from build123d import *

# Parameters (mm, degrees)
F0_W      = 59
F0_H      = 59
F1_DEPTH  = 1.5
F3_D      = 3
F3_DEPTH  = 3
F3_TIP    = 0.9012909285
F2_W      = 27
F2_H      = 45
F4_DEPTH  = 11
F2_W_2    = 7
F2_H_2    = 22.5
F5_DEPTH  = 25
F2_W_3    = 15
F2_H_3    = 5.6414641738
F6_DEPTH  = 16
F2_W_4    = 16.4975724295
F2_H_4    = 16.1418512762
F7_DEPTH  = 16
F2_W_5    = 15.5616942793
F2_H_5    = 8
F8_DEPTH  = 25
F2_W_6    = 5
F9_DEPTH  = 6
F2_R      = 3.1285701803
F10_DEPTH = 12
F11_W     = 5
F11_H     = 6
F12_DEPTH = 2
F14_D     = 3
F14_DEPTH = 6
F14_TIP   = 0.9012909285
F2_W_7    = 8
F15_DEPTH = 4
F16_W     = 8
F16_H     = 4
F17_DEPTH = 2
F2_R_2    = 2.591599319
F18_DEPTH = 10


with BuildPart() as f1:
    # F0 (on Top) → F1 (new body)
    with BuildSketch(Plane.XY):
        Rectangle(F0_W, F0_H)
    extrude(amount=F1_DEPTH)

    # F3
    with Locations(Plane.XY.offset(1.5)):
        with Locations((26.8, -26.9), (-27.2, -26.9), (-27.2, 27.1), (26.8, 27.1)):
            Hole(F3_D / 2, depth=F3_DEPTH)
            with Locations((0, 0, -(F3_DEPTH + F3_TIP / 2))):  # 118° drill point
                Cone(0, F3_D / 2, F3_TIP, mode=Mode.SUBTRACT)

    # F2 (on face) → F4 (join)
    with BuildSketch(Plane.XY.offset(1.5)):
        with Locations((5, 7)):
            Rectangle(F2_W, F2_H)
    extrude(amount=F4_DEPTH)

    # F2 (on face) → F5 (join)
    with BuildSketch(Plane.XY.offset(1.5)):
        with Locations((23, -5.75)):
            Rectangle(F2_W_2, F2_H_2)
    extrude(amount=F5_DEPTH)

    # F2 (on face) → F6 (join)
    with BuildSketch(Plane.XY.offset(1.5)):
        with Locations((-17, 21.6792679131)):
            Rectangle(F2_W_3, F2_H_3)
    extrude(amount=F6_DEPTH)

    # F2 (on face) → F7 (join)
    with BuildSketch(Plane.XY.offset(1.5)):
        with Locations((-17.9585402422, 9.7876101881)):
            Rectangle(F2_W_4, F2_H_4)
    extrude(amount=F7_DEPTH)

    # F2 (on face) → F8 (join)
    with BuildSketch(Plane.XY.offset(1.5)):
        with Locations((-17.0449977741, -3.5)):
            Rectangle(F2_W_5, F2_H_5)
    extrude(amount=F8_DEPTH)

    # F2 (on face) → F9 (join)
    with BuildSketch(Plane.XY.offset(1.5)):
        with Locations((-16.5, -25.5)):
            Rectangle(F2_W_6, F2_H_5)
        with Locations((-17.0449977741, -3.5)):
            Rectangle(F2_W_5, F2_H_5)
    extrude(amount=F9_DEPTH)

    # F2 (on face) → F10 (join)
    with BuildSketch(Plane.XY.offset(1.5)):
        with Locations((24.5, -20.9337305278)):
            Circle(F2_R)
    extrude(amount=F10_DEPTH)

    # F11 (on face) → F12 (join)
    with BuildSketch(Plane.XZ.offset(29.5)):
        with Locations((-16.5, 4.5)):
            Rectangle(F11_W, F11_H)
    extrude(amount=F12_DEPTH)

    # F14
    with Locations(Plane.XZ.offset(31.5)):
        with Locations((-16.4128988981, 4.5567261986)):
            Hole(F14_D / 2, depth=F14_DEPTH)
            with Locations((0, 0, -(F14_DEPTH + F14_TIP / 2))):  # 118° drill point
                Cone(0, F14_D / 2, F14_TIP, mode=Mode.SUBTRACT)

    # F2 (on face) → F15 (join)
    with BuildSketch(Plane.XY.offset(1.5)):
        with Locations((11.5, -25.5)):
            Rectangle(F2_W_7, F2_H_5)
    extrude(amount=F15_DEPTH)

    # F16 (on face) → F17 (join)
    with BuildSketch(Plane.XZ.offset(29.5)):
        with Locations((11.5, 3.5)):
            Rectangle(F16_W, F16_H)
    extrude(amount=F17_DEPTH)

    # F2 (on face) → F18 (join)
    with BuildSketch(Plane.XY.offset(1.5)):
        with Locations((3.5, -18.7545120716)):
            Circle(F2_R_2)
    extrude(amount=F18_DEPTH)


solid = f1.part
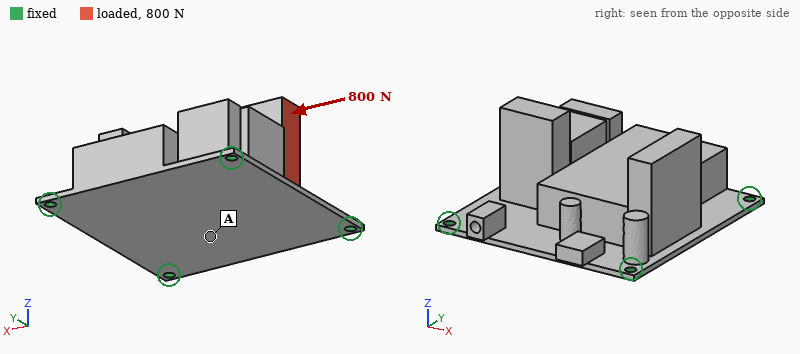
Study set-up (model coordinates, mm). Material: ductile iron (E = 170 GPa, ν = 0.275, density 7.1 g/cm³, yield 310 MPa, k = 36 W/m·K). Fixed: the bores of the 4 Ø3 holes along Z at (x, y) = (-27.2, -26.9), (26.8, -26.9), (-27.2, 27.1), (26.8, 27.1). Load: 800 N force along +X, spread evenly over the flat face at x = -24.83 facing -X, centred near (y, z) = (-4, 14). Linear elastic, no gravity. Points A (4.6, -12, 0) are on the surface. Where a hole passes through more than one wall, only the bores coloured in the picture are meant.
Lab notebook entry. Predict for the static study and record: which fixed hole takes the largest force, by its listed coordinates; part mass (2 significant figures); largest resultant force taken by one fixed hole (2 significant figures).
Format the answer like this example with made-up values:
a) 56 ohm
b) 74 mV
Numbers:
a) (26.8, 27.1)
b) 230 g
c) 430 N
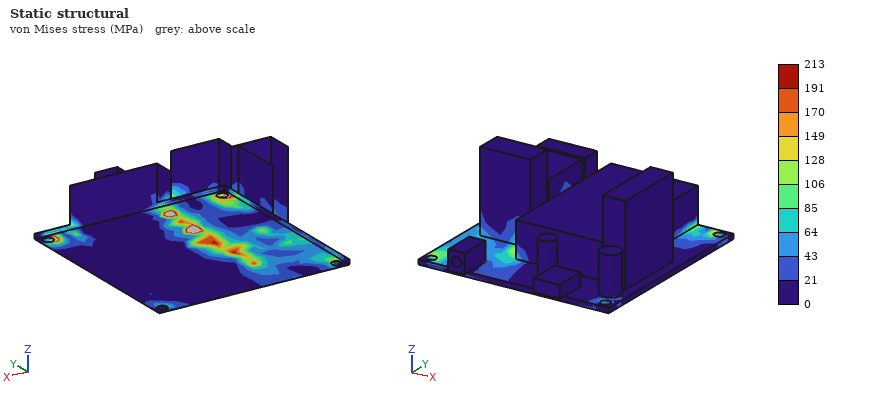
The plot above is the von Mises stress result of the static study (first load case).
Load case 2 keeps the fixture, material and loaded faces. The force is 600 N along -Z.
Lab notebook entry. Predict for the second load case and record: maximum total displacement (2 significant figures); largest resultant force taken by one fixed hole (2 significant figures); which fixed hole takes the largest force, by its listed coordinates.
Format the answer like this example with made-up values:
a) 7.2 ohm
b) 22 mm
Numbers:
a) 0.13 mm
b) 530 N
c) (-27.2, 27.1)
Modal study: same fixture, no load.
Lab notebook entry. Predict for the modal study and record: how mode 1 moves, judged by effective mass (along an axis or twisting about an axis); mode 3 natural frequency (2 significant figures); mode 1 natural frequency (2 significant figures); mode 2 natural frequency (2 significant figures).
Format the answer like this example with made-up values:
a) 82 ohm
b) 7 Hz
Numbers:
a) along Z
b) 2100 Hz
c) 1200 Hz
d) 1900 Hz
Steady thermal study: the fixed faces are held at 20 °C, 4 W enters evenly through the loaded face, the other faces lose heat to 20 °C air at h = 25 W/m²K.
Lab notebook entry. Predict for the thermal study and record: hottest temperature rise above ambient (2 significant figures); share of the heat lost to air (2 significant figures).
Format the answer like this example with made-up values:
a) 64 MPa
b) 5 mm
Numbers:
a) 27 K
b) 61 %
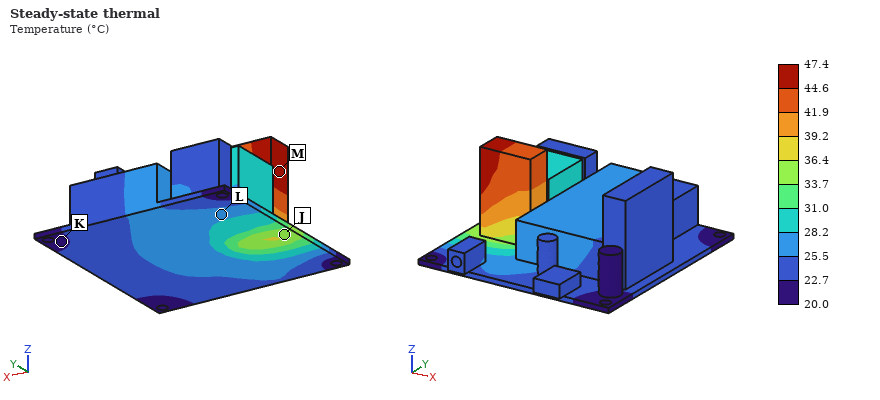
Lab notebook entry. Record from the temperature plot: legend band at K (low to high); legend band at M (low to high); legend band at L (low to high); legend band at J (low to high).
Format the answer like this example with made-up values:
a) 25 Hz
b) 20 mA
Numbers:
a) 20.0 to 22.7 °C
b) 44.6 to 47.4 °C
c) 25.5 to 28.2 °C
d) 33.7 to 36.4 °C
